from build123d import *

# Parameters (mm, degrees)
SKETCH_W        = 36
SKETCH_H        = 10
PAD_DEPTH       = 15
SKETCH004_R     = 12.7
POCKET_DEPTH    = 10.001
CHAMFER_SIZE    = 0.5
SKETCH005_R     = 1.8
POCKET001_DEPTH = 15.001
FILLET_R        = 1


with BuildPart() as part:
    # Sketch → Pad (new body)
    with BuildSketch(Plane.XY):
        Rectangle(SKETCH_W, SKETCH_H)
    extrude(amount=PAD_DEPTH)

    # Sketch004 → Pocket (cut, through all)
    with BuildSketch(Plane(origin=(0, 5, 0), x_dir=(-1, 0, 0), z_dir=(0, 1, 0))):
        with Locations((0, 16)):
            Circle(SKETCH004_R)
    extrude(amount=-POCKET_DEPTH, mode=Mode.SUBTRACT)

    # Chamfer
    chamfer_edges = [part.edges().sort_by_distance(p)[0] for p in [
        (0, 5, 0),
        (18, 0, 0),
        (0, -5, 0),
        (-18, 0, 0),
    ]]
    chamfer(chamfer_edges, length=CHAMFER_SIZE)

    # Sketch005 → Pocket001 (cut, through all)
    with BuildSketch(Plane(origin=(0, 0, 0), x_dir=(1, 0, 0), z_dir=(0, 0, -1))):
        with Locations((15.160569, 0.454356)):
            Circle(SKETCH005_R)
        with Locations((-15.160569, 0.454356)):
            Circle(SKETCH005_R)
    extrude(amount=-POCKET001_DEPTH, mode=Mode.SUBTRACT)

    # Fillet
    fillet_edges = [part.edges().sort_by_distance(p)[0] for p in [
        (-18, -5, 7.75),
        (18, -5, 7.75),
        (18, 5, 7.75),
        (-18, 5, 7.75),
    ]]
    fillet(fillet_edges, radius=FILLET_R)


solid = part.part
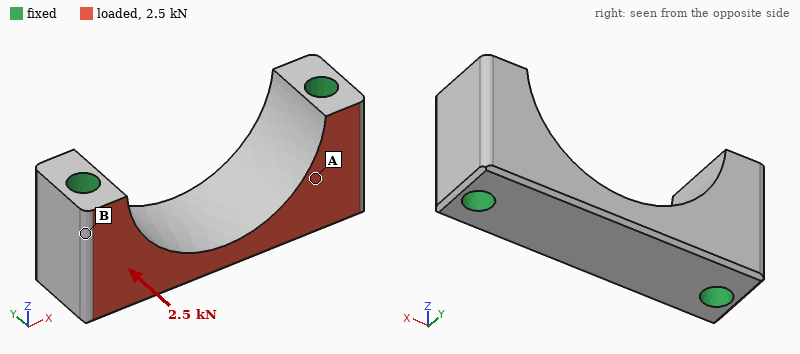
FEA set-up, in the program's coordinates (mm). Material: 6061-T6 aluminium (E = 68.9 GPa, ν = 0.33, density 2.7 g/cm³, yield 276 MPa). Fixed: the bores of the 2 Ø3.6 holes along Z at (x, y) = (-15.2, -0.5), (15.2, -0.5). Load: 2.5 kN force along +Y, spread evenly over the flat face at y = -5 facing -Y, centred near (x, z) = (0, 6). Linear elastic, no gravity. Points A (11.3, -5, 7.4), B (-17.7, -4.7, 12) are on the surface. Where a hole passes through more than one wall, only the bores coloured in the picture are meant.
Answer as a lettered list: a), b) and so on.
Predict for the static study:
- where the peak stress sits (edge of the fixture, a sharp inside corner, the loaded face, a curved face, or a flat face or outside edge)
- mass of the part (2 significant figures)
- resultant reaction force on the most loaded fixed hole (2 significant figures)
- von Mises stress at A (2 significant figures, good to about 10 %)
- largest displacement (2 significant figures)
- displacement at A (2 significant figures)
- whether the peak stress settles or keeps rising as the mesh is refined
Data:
a) edge of the fixture
b) 7.5 g
c) 1.3 kN
d) 16 MPa
e) 7.4 µm
f) 2.5 µm
g) keeps rising
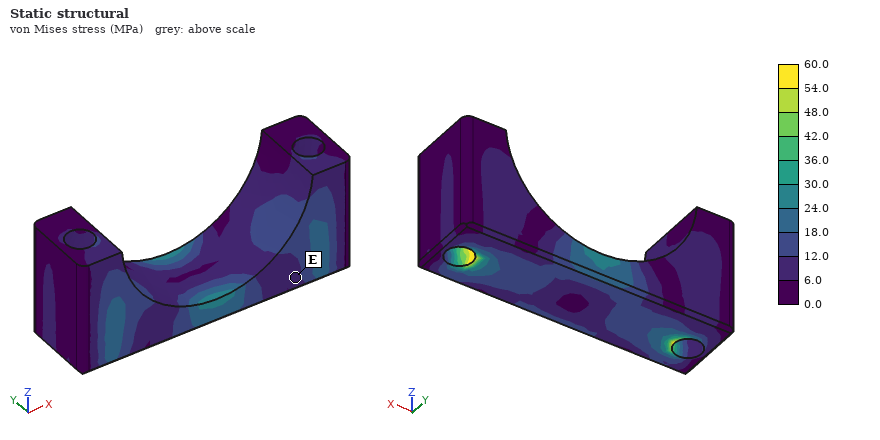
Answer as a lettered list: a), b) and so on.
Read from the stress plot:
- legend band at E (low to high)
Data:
a) 6.0 to 12.0 MPa
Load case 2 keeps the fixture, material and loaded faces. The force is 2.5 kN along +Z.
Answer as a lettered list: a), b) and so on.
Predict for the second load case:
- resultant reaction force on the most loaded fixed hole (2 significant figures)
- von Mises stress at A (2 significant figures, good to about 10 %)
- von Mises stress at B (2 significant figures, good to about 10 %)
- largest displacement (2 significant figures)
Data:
a) 1.3 kN
b) 31 MPa
c) 7.9 MPa
d) 13 µm
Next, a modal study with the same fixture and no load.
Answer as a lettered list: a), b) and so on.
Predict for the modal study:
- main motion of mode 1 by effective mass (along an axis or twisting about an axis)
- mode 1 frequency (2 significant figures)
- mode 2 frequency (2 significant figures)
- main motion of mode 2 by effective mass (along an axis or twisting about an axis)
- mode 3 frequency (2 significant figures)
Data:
a) along Y
b) 39 kHz
c) 46 kHz
d) along Z
e) 69 kHz
